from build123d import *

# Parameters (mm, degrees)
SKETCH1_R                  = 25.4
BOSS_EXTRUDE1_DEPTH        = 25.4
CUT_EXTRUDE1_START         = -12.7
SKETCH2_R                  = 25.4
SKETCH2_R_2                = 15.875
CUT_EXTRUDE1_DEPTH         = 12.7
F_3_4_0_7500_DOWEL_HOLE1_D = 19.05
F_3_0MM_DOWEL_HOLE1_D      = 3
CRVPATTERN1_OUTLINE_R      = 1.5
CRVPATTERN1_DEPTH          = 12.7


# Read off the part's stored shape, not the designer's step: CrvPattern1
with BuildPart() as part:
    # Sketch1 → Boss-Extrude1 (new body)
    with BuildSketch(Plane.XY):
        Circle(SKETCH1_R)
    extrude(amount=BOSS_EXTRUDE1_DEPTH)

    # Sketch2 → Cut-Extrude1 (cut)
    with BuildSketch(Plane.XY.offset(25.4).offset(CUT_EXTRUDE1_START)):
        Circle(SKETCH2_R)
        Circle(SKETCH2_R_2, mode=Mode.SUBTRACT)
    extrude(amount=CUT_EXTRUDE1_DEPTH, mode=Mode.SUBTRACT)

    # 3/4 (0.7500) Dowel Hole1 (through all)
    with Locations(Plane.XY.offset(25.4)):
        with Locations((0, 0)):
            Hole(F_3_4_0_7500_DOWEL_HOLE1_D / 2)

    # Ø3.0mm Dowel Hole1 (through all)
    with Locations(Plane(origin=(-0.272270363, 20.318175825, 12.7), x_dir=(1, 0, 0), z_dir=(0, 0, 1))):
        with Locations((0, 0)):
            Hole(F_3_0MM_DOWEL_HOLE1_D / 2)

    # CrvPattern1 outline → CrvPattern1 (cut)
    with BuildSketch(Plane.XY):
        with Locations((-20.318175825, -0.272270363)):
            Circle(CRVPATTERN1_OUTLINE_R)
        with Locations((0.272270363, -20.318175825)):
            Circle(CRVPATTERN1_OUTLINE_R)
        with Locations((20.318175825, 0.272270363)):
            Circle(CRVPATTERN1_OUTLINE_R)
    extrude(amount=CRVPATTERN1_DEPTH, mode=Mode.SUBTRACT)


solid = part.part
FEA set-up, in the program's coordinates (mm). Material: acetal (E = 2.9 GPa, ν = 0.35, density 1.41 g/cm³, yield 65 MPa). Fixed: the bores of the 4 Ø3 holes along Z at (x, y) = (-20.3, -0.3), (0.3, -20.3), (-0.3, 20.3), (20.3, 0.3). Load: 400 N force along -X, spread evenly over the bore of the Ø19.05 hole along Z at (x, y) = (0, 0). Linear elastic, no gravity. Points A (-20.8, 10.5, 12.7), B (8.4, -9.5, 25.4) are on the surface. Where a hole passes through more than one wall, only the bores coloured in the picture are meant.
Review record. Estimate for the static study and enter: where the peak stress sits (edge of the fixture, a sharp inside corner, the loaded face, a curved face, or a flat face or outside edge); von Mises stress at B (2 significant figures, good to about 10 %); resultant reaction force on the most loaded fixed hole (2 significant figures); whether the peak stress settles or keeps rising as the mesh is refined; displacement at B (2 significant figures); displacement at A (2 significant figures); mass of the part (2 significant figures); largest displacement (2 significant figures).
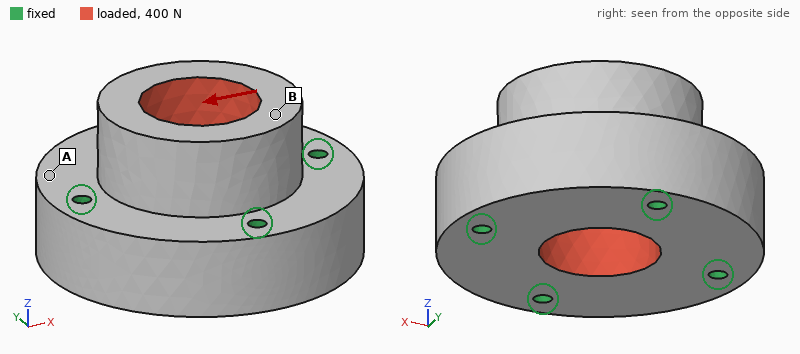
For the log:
edge of the fixture
0.42 MPa
130 N
keeps rising
10 µm
3.4 µm
40 g
12 µm
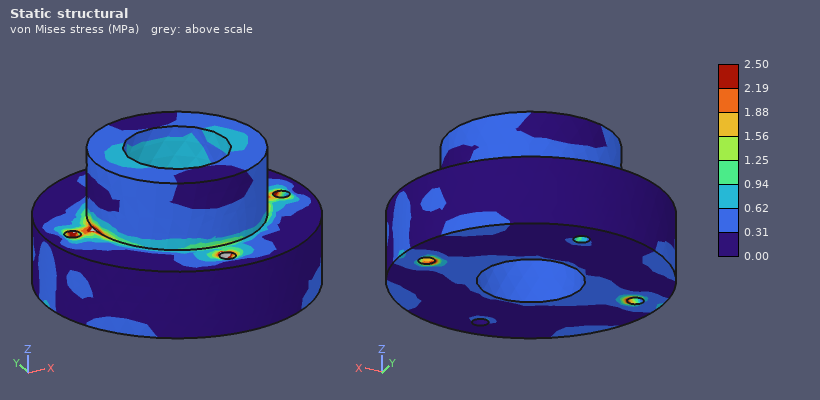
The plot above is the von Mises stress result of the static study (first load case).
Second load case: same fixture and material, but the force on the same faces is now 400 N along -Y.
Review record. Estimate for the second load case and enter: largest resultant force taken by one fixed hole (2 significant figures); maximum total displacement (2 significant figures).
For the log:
130 N
12 µm
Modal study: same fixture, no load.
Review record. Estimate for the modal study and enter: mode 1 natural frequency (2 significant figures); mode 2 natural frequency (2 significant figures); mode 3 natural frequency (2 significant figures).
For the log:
7700 Hz
7700 Hz
8200 Hz
